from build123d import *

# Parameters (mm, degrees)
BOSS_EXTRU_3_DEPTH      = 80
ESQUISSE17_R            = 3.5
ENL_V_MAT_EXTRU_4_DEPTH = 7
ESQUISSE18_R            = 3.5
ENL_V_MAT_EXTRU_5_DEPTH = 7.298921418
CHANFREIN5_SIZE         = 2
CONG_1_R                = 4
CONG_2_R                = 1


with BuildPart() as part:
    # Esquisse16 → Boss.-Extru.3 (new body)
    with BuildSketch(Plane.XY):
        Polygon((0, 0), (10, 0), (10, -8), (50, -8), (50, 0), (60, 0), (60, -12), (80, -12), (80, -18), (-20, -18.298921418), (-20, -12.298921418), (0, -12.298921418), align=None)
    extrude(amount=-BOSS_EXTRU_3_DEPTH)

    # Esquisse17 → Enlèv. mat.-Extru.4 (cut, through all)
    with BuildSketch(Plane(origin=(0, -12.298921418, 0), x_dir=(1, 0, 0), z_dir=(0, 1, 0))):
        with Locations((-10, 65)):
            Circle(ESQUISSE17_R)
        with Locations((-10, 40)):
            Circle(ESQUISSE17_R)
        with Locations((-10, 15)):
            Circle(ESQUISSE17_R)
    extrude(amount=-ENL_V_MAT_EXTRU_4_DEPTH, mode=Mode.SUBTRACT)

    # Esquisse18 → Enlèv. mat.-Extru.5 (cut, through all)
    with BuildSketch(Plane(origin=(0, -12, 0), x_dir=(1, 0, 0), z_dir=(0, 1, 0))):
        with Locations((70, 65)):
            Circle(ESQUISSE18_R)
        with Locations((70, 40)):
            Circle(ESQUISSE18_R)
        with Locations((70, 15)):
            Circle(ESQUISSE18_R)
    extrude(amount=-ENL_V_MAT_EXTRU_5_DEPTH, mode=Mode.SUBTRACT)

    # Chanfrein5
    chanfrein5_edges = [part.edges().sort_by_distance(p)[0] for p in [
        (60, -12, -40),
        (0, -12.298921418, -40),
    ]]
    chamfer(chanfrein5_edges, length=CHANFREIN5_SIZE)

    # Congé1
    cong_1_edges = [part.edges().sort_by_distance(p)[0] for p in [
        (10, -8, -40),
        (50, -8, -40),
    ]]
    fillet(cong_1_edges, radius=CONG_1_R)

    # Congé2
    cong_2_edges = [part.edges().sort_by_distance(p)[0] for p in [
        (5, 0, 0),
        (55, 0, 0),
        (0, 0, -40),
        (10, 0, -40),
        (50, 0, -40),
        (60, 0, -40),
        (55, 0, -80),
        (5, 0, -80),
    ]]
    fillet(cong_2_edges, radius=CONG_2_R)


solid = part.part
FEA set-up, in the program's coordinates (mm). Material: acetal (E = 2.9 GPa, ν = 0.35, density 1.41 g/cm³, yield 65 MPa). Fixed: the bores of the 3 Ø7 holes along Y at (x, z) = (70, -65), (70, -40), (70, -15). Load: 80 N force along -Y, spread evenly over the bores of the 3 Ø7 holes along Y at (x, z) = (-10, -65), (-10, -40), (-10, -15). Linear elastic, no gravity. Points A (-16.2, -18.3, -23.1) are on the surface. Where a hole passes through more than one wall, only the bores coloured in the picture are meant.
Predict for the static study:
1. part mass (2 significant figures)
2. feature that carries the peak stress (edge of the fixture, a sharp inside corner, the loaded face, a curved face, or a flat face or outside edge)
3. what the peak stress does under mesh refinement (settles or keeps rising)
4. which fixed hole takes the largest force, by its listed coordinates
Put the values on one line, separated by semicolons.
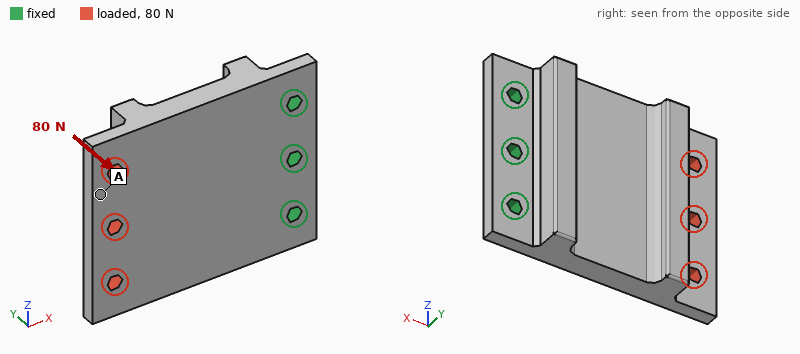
110 g; edge of the fixture; keeps rising; (70, -40)
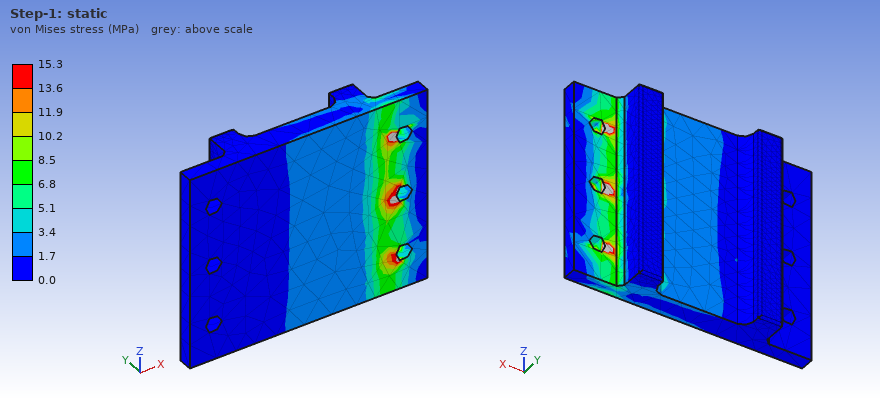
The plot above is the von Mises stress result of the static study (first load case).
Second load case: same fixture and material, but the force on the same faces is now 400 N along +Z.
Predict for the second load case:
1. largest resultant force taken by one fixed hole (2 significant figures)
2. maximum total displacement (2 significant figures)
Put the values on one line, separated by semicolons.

600 N; 0.24 mm
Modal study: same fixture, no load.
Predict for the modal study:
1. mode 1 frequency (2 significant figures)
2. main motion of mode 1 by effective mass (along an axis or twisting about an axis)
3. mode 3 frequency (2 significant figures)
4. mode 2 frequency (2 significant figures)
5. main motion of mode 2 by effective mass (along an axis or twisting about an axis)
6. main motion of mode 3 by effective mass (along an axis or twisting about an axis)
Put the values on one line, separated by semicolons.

210 Hz; along Y; 1300 Hz; 700 Hz; twisting about X; along Z
